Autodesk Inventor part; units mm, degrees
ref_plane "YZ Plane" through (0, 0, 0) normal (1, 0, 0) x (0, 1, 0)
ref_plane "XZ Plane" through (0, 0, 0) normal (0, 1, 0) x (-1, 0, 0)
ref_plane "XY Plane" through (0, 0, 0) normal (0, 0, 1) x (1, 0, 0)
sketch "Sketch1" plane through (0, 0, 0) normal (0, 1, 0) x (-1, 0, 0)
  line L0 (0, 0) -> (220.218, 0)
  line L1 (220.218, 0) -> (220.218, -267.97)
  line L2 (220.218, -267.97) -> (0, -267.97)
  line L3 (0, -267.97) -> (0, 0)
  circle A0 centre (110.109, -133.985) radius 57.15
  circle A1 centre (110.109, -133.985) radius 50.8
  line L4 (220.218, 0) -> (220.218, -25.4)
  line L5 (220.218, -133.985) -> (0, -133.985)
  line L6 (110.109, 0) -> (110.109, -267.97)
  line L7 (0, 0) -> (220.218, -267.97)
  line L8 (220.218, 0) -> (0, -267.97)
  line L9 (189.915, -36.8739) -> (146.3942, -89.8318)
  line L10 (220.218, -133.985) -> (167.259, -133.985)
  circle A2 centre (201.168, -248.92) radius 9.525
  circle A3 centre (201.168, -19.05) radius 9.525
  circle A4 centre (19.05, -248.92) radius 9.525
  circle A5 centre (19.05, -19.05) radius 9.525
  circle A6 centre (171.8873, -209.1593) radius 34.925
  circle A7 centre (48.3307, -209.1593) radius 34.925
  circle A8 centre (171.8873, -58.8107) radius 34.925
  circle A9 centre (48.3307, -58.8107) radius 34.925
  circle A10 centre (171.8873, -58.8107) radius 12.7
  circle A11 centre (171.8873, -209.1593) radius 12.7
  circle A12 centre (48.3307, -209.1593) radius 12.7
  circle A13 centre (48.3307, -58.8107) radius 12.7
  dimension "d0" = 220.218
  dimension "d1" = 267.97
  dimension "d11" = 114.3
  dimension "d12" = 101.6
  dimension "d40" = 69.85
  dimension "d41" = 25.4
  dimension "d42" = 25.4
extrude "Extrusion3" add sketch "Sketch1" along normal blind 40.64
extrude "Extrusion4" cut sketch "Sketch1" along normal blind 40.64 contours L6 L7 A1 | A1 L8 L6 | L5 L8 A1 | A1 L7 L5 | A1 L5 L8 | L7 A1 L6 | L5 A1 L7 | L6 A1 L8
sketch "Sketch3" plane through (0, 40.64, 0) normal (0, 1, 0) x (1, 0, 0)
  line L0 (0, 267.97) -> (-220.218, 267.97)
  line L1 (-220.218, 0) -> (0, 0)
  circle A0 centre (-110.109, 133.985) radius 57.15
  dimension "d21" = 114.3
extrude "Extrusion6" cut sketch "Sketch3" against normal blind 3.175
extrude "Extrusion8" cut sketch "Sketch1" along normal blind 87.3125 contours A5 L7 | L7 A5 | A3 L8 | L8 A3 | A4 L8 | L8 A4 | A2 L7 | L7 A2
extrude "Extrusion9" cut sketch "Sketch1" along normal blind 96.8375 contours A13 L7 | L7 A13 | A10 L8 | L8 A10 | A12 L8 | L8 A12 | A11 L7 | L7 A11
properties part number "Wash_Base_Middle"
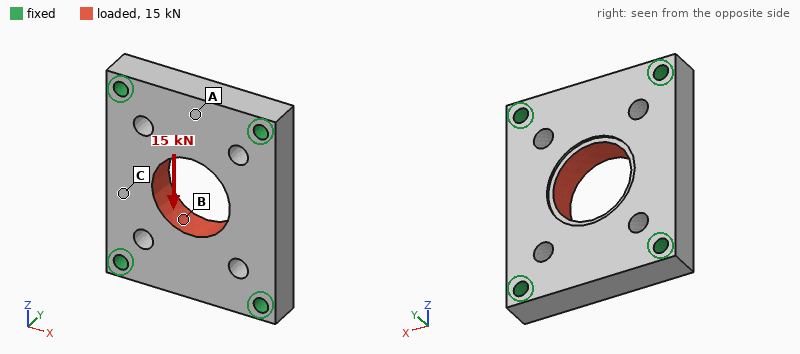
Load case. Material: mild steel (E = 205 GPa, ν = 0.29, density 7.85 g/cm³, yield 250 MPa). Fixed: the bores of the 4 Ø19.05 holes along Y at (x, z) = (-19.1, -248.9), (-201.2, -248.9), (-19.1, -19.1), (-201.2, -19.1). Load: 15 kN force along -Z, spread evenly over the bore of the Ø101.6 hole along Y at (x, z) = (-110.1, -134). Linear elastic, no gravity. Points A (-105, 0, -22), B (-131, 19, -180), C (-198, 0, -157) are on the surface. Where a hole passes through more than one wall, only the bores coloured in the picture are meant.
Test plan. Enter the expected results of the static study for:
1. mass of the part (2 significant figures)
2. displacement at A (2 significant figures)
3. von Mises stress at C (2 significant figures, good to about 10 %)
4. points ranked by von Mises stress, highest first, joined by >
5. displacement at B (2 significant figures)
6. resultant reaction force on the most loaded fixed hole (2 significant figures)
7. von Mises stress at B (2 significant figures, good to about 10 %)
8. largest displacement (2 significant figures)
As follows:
15 kg
1.0 µm
0.85 MPa
B > C > A
1.1 µm
4.0 kN
1.3 MPa
1.2 µm
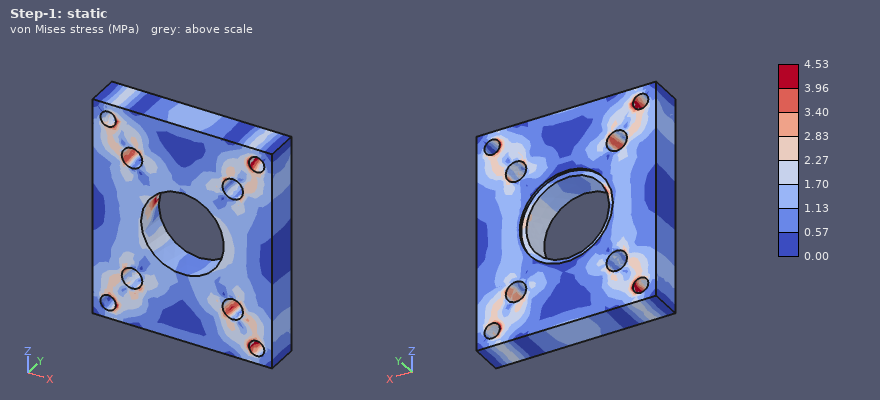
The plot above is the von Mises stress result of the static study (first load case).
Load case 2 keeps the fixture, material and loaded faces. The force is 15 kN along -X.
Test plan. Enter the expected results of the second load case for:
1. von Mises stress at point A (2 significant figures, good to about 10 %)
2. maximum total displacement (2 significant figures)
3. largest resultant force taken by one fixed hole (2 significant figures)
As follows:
0.85 MPa
1.8 µm
4.2 kN
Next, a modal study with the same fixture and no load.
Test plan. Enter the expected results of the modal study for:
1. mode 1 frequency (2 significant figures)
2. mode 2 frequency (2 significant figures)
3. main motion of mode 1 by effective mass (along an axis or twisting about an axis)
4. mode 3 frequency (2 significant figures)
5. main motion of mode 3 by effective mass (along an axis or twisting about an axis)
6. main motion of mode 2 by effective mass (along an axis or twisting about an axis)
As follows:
2900 Hz
3800 Hz
along Y
4700 Hz
twisting about X
twisting about Z
